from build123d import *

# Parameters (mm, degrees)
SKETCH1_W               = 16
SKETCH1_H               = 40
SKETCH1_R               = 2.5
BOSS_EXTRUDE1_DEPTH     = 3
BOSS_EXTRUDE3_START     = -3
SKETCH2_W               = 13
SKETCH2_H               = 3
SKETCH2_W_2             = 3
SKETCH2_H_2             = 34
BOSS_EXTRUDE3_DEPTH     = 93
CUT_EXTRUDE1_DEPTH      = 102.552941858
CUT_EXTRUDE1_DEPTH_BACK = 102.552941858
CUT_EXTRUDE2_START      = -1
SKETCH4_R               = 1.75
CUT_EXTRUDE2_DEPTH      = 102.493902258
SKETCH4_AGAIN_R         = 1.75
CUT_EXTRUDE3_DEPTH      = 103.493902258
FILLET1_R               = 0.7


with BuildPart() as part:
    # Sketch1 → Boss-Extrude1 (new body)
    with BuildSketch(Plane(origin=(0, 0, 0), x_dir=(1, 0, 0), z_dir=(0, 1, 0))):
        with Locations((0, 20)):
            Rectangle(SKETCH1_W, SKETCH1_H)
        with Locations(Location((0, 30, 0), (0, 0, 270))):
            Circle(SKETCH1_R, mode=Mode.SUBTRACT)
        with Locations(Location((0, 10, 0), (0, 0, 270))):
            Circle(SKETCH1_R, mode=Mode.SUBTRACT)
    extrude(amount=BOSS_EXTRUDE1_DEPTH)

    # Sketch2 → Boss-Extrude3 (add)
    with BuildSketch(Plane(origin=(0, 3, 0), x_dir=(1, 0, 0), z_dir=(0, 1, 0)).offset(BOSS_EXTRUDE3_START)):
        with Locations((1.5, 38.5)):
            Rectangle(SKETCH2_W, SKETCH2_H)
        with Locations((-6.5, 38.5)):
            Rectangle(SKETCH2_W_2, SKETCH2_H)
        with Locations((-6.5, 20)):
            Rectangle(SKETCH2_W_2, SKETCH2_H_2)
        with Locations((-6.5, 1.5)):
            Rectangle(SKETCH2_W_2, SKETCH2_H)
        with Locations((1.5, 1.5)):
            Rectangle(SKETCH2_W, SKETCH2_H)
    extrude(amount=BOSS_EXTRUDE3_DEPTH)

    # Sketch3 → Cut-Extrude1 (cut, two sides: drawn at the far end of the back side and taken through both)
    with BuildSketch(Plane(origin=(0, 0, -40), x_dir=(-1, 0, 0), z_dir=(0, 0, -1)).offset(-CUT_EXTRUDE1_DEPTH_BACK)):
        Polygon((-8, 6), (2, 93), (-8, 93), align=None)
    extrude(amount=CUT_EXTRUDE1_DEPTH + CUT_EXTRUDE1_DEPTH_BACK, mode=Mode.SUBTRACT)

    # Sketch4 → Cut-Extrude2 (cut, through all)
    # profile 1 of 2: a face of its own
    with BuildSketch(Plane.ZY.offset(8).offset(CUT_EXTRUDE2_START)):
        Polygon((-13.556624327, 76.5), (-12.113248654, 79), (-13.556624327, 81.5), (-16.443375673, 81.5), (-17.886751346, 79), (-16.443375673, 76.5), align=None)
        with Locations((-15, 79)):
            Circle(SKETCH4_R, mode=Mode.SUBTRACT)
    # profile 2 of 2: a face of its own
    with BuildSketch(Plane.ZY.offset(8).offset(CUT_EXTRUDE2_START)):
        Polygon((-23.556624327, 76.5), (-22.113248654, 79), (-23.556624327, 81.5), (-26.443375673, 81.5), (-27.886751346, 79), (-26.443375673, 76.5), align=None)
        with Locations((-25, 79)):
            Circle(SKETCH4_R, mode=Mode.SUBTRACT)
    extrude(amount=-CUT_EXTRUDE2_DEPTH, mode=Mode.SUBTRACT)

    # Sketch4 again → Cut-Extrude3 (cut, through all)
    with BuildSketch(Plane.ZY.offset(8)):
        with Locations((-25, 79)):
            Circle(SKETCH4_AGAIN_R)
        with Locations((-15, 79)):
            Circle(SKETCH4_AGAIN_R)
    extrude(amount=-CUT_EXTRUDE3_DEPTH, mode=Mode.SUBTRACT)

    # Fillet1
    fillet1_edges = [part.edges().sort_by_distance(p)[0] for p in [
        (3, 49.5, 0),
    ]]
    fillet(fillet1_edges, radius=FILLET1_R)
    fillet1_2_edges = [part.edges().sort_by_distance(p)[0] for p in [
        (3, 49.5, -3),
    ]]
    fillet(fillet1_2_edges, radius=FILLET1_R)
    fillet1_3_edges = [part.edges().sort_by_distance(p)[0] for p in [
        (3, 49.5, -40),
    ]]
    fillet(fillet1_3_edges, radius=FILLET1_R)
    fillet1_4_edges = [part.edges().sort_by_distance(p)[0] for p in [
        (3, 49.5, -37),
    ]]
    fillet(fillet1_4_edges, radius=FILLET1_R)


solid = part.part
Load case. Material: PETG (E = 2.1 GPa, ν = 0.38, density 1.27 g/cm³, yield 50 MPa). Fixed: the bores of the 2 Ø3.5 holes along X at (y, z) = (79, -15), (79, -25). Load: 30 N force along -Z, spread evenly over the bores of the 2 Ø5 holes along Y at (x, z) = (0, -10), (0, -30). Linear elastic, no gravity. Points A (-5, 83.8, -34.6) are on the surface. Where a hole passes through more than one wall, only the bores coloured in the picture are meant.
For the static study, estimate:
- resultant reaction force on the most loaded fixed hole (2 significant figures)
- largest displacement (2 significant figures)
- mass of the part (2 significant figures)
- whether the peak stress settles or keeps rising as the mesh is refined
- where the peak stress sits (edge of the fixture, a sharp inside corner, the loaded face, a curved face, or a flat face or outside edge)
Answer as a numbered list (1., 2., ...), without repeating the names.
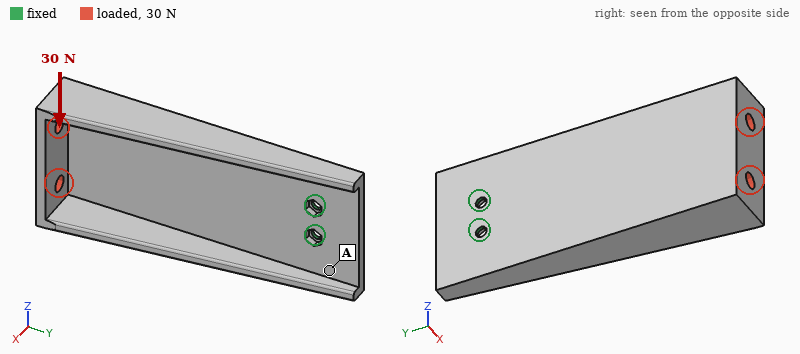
1. 200 N
2. 1.1 mm
3. 21 g
4. keeps rising
5. edge of the fixture
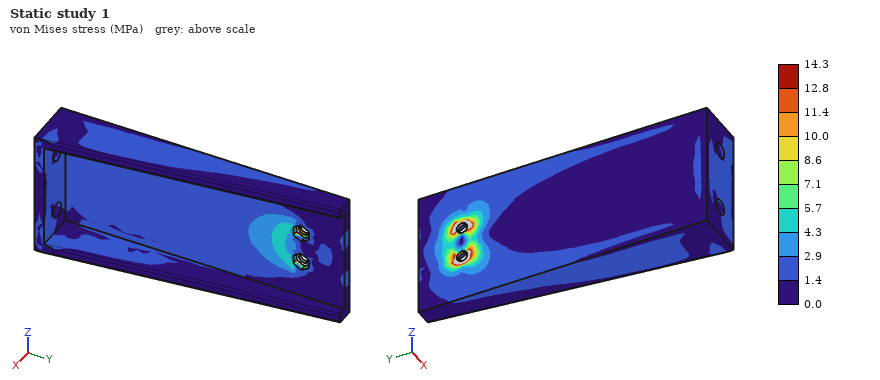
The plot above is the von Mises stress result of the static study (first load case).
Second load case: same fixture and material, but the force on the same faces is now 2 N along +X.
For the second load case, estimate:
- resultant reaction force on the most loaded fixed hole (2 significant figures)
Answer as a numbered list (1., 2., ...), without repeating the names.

1. 1.4 N
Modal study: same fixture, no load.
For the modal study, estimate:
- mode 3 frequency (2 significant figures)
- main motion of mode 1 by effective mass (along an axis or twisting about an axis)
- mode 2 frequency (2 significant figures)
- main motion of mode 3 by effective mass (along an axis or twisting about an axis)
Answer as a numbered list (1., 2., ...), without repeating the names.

1. 400 Hz
2. along X
3. 270 Hz
4. along Z
